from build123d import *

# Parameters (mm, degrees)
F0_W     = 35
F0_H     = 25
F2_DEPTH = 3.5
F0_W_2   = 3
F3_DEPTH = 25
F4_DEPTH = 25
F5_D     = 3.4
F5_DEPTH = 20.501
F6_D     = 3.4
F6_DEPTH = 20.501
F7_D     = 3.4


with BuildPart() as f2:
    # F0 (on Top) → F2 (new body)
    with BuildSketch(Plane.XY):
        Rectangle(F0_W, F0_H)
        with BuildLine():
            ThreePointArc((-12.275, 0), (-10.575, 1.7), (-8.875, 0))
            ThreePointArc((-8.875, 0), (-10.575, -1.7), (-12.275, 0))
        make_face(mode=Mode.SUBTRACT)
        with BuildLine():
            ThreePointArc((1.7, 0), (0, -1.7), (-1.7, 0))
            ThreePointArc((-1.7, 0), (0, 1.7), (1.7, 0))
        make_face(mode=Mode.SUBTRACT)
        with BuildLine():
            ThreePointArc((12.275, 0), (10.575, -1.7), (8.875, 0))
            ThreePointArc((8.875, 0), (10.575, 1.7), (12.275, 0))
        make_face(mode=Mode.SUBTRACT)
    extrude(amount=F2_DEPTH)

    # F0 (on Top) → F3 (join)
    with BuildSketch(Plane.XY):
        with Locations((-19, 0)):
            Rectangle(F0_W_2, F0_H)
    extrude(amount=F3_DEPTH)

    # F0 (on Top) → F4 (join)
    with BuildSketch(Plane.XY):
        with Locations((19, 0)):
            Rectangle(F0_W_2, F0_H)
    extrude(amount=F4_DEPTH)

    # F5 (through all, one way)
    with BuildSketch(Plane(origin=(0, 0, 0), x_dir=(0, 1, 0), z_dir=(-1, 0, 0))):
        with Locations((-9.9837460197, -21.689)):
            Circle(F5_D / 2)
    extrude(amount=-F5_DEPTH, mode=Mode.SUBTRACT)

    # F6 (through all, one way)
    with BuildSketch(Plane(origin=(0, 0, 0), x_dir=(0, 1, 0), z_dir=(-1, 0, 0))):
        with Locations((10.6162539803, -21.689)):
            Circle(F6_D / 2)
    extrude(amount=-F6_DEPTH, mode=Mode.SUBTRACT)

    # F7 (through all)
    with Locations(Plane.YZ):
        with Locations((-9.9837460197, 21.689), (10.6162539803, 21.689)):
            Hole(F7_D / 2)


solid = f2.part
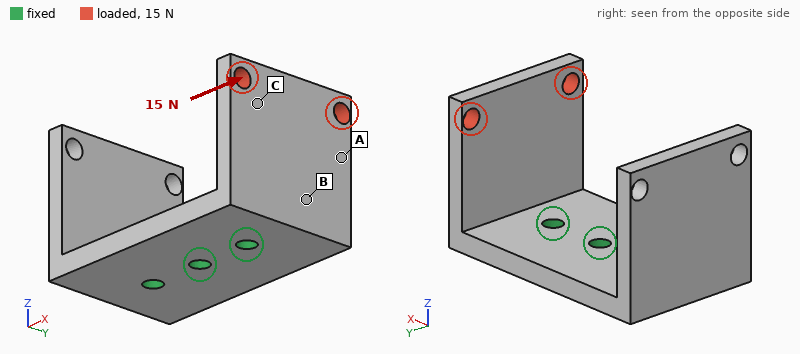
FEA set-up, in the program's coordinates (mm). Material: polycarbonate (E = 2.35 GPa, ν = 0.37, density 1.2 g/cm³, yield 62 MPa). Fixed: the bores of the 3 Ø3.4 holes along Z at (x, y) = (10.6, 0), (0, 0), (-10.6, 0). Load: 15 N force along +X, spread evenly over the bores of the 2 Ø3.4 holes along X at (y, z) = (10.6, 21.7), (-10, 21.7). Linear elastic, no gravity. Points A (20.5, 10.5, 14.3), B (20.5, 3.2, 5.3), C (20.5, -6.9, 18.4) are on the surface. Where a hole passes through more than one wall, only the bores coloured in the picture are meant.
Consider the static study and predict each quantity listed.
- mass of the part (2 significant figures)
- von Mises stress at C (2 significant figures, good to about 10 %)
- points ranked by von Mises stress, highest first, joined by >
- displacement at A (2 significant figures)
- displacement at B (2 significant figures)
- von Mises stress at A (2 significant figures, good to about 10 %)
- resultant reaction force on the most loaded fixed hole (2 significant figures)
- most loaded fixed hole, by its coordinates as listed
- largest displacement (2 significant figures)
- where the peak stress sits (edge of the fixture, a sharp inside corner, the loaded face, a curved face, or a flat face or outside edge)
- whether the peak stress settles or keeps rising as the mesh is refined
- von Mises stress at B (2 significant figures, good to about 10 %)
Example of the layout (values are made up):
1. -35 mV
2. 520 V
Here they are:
1. 7.9 g
2. 1.4 MPa
3. B > A > C
4. 0.28 mm
5. 0.096 mm
6. 3.2 MPa
7. 17 N
8. (10.6, 0)
9. 0.61 mm
10. edge of the fixture
11. keeps rising
12. 5.8 MPa
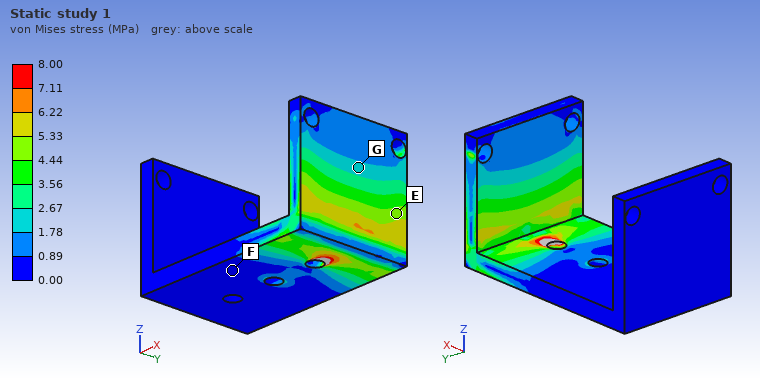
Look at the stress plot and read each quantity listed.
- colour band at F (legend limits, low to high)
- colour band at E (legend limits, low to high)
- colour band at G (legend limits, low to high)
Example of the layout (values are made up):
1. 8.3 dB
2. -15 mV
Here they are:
1. 0.00 to 0.89 MPa
2. 4.44 to 5.33 MPa
3. 1.78 to 2.67 MPa
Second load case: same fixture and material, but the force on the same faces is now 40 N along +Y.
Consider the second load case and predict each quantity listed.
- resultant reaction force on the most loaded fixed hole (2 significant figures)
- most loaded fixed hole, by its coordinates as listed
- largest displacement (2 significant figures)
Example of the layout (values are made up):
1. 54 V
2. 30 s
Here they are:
1. 53 N
2. (10.6, 0)
3. 0.59 mm
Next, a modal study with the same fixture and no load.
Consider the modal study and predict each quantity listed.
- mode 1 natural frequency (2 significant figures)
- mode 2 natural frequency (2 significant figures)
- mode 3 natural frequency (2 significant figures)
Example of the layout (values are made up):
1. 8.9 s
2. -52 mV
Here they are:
1. 970 Hz
2. 980 Hz
3. 1400 Hz
